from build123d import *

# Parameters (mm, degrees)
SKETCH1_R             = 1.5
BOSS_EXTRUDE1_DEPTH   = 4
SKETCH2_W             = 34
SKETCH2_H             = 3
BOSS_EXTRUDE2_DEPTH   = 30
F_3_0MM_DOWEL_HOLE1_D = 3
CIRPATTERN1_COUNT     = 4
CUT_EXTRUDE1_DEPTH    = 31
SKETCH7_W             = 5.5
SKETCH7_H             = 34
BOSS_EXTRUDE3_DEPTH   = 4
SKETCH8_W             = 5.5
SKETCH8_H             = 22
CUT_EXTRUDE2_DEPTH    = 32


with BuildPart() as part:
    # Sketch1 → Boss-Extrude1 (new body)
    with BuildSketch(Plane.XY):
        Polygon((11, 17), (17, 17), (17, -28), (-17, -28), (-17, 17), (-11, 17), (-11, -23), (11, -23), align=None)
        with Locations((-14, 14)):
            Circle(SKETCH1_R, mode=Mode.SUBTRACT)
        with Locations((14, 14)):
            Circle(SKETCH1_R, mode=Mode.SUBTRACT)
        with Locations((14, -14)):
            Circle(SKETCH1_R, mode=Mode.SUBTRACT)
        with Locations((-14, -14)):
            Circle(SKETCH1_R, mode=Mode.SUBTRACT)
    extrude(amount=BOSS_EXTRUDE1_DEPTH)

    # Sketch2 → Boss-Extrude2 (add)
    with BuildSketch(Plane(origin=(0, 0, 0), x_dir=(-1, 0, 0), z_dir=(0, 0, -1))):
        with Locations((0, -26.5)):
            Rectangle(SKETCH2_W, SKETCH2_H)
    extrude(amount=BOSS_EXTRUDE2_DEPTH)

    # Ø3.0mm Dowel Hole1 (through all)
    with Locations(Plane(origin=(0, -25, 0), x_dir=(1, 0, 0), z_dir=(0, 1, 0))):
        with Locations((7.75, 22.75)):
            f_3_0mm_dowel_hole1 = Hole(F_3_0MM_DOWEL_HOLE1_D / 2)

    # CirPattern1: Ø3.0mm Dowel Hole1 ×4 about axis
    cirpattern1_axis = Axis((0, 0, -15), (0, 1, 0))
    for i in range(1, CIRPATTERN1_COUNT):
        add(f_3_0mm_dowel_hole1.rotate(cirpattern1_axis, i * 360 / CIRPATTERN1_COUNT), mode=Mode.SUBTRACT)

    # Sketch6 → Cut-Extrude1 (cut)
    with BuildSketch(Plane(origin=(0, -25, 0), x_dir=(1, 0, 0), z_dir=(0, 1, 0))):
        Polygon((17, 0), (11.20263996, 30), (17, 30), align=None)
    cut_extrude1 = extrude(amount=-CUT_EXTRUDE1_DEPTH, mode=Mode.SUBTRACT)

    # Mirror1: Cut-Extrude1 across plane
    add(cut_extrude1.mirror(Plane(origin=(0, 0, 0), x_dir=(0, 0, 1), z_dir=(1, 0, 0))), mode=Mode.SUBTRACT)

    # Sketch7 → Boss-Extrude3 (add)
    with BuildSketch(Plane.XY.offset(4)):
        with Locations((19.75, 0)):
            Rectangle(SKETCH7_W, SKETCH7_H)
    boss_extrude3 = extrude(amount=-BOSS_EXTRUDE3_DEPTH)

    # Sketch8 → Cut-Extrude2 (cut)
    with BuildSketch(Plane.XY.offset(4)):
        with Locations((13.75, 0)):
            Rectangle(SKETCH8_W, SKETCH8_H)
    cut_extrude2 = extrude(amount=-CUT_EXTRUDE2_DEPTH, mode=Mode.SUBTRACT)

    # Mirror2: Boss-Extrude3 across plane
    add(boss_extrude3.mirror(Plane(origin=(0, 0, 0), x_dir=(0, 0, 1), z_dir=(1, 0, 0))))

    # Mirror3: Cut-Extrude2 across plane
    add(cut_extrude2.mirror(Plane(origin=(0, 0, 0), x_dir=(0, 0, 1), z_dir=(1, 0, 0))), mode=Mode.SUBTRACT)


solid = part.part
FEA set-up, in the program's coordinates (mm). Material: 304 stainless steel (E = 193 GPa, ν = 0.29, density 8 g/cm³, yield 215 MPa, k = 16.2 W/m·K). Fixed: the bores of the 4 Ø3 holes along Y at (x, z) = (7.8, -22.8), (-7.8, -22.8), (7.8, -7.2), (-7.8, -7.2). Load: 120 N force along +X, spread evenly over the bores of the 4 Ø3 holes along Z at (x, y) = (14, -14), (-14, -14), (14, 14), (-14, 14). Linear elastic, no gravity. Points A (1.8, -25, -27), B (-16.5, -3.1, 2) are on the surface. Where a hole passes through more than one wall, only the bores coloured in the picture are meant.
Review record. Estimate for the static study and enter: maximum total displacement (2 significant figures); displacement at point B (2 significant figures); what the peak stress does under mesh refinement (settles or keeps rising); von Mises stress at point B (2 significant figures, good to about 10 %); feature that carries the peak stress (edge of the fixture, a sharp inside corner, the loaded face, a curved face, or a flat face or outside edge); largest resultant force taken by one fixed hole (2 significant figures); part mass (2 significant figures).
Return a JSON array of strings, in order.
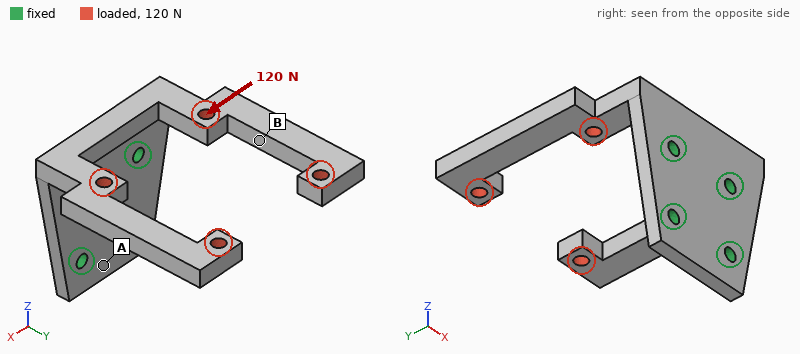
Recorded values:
["0.12 mm", "0.051 mm", "keeps rising", "21 MPa", "edge of the fixture", "170 N", "44 g"]
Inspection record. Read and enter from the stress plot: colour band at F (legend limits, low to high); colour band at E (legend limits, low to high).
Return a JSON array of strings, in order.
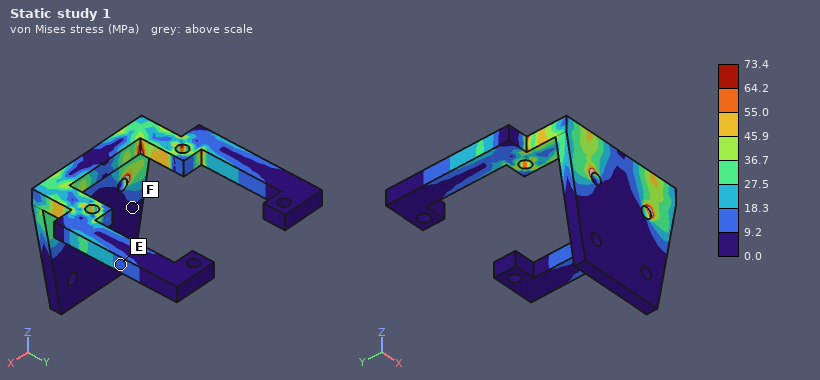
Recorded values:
["0.0 to 9.2 MPa", "9.2 to 18.3 MPa"]
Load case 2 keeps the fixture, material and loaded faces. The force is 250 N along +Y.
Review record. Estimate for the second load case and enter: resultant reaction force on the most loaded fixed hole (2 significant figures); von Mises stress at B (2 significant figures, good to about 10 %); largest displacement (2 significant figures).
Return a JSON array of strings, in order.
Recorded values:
["140 N", "17 MPa", "39 µm"]
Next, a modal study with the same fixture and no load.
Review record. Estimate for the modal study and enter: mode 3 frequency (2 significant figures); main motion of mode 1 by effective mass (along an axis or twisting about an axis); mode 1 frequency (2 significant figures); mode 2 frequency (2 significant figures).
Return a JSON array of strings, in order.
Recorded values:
["1500 Hz", "along Z", "1100 Hz", "1100 Hz"]
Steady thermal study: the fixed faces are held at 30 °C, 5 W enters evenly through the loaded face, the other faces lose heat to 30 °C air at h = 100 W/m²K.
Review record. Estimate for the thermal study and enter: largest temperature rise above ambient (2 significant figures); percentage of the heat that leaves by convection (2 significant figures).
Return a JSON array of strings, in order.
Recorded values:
["39 K", "88 %"]
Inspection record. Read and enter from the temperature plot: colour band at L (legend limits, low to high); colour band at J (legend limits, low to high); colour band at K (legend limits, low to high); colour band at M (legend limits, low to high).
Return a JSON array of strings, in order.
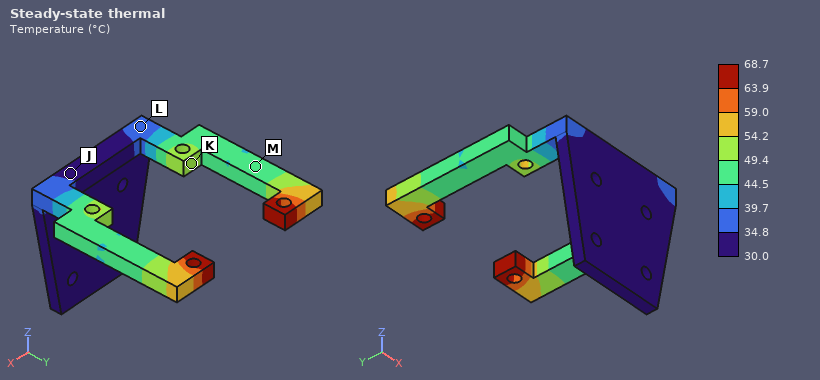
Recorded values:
["34.8 to 39.7 °C", "30.0 to 34.8 °C", "49.4 to 54.2 °C", "44.5 to 49.4 °C"]
